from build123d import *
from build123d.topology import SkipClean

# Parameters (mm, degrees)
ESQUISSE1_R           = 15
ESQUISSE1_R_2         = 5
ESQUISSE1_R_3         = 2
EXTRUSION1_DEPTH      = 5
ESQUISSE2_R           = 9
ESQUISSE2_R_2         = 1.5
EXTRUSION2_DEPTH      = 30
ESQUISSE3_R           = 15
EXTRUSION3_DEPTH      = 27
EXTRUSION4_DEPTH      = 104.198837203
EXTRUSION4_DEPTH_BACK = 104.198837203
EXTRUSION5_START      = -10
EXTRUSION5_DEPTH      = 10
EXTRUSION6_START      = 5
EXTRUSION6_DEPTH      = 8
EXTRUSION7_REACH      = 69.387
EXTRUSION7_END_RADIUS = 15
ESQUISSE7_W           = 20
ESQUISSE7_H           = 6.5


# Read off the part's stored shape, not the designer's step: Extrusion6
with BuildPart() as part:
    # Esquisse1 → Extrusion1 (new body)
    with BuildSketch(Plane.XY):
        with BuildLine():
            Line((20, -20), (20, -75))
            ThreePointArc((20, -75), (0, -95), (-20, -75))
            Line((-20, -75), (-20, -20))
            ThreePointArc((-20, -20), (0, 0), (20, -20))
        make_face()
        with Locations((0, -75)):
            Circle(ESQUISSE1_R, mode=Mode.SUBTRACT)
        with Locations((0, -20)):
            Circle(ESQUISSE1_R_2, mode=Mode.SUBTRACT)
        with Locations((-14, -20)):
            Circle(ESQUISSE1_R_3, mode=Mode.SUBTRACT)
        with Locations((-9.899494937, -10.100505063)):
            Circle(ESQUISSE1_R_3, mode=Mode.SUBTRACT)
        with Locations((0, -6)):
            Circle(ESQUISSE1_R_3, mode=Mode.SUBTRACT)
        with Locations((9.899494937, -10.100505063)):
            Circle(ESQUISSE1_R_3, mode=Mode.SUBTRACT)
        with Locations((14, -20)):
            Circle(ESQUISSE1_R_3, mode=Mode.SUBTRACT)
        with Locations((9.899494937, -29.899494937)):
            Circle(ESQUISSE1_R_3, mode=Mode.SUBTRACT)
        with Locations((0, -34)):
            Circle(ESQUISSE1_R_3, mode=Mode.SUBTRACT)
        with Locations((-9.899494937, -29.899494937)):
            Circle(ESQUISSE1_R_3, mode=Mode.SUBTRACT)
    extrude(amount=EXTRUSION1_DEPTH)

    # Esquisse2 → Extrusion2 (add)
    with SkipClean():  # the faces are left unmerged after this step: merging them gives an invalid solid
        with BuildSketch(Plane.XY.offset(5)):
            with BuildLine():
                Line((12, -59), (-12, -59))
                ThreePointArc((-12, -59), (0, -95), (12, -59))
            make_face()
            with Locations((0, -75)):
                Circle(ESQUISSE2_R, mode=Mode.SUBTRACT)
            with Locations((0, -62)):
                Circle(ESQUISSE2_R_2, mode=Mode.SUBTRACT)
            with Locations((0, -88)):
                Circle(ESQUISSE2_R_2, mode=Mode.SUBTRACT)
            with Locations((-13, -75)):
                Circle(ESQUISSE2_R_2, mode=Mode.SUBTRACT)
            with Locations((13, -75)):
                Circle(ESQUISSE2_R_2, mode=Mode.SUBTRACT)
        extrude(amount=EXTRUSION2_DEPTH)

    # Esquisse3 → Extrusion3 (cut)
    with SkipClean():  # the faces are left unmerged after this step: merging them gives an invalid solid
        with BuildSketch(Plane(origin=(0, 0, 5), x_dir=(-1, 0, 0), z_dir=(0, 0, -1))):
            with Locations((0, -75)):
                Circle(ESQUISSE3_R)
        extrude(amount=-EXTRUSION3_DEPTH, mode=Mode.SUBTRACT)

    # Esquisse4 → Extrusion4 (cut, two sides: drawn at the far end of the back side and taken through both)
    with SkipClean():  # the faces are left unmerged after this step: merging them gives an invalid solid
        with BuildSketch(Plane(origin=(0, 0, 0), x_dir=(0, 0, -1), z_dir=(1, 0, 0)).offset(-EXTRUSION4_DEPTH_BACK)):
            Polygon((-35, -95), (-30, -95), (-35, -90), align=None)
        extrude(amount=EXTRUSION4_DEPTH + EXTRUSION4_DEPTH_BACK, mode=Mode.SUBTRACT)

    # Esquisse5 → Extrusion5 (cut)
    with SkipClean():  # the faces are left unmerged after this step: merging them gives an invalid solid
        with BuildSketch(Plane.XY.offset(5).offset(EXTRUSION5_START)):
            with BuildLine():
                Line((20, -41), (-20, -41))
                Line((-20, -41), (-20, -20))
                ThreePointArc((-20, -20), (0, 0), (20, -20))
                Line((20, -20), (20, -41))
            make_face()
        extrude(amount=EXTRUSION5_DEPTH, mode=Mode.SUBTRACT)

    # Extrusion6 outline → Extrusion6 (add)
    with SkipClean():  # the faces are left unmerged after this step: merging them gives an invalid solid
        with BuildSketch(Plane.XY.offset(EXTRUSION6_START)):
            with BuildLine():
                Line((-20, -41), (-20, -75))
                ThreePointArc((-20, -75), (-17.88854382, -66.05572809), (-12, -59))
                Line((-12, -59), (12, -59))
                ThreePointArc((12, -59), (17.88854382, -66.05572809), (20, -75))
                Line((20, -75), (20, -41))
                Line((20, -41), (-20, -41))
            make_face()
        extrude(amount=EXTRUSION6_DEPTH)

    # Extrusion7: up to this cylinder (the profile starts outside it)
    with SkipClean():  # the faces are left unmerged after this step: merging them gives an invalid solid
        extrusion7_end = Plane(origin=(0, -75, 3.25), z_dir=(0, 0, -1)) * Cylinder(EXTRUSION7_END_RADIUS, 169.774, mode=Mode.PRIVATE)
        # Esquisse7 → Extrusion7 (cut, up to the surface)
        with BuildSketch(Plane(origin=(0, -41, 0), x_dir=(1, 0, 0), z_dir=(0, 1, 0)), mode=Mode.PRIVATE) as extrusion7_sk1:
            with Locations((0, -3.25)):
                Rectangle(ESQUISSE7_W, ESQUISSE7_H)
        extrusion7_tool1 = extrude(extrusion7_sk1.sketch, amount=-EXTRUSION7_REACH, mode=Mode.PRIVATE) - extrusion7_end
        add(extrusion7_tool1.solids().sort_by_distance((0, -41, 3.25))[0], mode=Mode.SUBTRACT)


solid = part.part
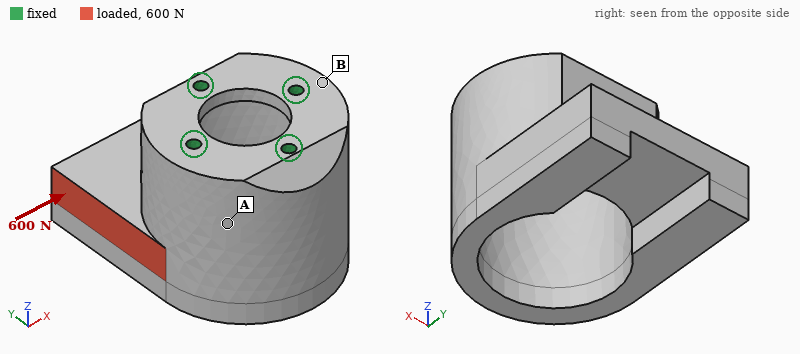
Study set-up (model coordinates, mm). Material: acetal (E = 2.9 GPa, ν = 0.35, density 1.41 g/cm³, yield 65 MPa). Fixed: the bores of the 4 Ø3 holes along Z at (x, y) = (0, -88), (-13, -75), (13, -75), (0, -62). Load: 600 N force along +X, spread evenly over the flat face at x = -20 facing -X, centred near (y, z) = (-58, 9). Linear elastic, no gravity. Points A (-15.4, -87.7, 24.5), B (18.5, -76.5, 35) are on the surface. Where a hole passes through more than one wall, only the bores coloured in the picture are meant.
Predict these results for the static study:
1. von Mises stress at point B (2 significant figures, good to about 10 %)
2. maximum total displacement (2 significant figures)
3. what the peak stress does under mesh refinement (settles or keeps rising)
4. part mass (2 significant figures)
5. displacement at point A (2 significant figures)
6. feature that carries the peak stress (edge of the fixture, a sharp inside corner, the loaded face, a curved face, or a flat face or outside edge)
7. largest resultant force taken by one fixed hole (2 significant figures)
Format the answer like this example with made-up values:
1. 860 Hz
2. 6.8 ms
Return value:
1. 10 MPa
2. 0.49 mm
3. keeps rising
4. 36 g
5. 0.13 mm
6. edge of the fixture
7. 510 N
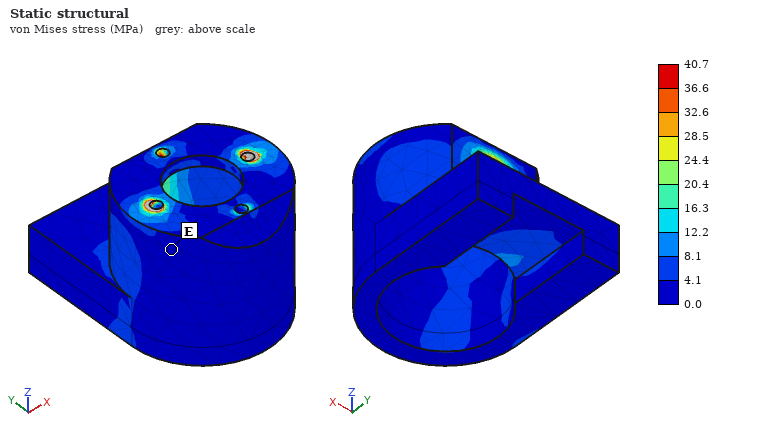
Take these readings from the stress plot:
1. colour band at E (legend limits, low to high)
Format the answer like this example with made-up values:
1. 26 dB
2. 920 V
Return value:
1. 0.0 to 4.1 MPa
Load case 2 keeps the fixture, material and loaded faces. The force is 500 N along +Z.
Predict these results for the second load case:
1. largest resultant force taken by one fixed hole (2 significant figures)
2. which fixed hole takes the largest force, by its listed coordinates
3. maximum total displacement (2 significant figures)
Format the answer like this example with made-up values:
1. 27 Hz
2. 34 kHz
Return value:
1. 500 N
2. (-13, -75)
3. 0.80 mm
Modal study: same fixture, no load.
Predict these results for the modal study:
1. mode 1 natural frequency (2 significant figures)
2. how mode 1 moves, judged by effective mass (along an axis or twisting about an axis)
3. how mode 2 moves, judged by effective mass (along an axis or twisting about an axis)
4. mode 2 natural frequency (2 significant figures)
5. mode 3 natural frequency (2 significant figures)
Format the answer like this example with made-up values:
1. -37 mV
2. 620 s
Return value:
1. 1200 Hz
2. along Y
3. along X
4. 1300 Hz
5. 2500 Hz
